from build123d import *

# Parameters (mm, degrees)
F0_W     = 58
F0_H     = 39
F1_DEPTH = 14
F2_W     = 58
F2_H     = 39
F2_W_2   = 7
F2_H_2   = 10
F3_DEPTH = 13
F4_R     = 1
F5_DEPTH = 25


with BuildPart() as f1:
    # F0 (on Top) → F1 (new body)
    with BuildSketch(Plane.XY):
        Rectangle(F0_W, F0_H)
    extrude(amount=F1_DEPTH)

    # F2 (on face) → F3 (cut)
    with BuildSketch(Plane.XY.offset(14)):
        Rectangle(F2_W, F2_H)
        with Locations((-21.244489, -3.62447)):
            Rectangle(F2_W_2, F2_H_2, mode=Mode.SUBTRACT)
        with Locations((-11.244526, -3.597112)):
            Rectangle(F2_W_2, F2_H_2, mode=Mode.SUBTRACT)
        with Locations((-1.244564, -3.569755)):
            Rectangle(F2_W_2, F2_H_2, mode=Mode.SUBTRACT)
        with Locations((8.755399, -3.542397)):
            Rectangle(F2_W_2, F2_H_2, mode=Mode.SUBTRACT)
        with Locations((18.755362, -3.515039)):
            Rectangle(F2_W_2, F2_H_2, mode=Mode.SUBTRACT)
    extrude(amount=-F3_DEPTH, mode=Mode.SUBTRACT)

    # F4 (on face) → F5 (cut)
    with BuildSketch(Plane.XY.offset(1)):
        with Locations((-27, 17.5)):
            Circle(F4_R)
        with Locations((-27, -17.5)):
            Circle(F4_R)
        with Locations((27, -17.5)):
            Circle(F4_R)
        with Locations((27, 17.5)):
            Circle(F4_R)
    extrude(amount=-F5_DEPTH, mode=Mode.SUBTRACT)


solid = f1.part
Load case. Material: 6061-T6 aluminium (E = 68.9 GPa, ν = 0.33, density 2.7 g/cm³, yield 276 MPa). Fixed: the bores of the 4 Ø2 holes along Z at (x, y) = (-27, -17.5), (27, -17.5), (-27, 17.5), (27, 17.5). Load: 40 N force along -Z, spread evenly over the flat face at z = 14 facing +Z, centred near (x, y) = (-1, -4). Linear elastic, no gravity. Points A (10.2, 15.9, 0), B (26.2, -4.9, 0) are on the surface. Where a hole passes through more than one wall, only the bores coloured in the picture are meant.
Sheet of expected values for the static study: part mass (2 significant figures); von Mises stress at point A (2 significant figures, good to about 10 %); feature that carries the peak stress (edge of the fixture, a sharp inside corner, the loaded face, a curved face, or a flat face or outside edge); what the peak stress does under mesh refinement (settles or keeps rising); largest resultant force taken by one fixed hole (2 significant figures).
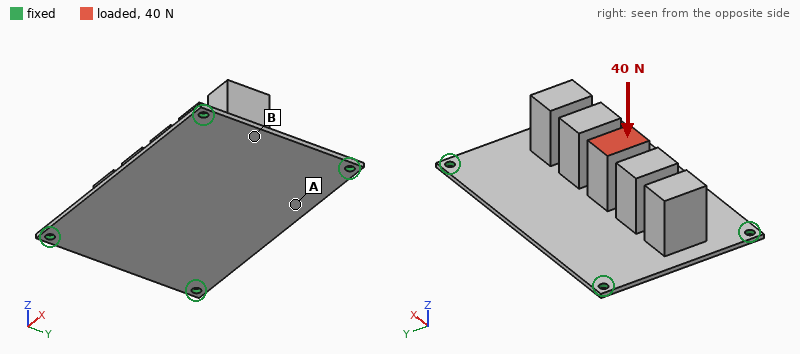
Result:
18 g
13 MPa
edge of the fixture
keeps rising
15 N
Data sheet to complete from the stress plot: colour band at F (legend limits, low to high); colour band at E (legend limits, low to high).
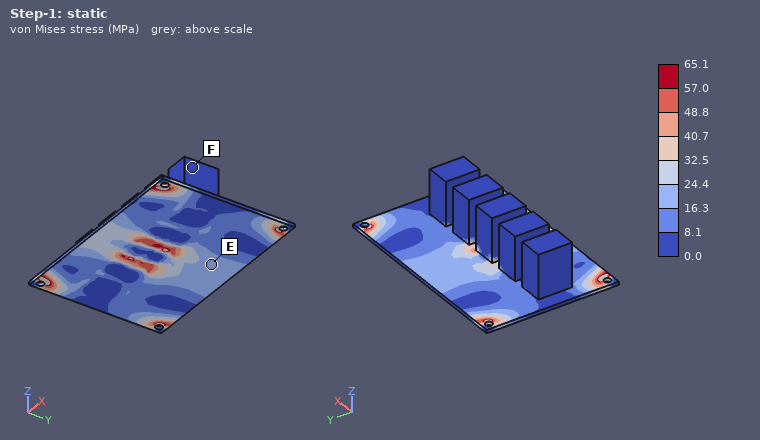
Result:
0.0 to 8.1 MPa
16.3 to 24.4 MPa
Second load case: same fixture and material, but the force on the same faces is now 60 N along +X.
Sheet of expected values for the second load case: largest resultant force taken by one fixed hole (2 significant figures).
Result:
24 N
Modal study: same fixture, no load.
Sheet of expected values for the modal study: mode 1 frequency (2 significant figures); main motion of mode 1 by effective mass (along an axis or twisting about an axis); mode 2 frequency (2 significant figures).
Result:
800 Hz
along Z
1800 Hz
